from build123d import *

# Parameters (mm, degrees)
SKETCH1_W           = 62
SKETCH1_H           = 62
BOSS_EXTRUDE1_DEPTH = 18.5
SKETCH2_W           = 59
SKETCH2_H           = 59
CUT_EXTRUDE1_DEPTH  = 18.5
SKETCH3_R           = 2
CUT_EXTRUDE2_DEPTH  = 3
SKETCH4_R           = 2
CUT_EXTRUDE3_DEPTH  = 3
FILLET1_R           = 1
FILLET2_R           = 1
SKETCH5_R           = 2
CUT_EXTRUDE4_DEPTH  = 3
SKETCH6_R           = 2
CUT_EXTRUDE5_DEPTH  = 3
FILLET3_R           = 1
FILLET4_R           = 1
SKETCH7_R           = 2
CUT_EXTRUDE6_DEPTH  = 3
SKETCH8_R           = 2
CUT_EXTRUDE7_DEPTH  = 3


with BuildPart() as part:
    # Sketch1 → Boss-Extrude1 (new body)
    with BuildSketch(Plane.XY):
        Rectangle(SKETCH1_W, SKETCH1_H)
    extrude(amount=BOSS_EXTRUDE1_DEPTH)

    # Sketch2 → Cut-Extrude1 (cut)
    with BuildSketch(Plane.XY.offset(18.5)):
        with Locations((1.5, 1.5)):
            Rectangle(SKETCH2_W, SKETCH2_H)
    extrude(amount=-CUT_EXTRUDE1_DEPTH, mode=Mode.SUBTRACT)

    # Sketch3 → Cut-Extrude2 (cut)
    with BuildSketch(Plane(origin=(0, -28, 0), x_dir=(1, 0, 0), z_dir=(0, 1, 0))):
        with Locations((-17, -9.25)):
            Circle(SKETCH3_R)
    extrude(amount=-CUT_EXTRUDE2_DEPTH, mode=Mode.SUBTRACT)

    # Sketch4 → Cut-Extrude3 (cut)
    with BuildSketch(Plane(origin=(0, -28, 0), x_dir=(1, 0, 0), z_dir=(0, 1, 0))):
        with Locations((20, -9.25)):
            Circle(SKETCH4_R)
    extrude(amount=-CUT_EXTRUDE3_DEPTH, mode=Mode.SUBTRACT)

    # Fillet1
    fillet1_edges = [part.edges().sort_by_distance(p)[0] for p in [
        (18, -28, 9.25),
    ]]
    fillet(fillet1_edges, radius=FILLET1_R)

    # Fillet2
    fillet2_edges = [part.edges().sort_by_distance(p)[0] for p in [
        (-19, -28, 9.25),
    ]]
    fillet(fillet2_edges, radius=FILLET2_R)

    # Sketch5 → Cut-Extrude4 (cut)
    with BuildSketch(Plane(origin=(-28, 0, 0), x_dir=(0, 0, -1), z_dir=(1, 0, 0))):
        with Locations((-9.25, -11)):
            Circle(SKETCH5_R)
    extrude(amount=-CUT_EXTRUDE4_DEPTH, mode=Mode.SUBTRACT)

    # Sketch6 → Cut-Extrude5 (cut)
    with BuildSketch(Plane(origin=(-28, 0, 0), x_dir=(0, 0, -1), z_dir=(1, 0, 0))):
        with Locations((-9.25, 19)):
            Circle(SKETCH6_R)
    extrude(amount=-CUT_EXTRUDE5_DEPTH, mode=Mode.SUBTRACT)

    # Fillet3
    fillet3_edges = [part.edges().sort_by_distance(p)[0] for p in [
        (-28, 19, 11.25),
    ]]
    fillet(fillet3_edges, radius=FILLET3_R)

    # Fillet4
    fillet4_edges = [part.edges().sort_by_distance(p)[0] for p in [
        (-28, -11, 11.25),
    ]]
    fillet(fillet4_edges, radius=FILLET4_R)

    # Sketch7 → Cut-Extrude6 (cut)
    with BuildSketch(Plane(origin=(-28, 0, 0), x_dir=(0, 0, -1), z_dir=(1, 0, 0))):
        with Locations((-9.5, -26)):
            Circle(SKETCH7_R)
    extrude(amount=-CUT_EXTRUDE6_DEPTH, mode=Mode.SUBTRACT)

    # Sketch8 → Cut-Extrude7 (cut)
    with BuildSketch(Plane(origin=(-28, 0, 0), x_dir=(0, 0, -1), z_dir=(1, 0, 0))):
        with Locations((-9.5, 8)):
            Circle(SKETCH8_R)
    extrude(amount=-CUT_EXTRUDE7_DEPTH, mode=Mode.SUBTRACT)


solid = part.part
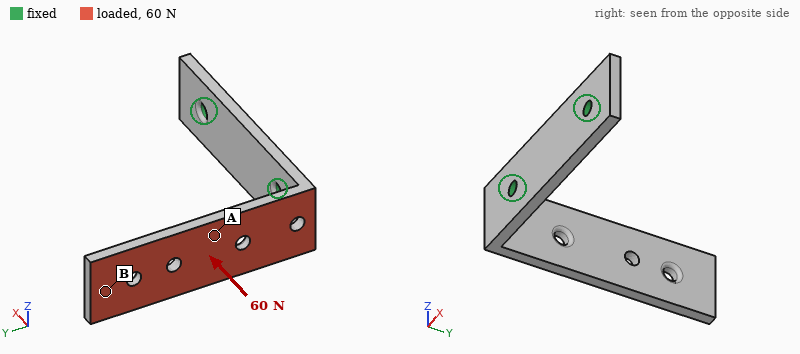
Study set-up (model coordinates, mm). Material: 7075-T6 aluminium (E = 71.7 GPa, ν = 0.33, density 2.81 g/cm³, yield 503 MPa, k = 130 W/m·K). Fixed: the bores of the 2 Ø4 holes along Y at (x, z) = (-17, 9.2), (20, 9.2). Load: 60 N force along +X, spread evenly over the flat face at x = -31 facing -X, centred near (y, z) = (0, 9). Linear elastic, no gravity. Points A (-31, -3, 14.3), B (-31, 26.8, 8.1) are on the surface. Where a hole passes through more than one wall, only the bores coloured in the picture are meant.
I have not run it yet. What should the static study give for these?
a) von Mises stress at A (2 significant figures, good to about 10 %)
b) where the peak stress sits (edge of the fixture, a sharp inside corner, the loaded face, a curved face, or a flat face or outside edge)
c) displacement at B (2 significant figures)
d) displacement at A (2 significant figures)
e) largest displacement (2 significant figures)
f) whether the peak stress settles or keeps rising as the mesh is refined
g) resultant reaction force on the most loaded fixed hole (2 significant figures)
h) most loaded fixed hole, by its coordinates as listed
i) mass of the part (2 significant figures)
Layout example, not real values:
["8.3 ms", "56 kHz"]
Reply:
["21 MPa", "edge of the fixture", "0.95 mm", "0.37 mm", "1.0 mm", "keeps rising", "42 N", "(20, 9.2)", "18 g"]
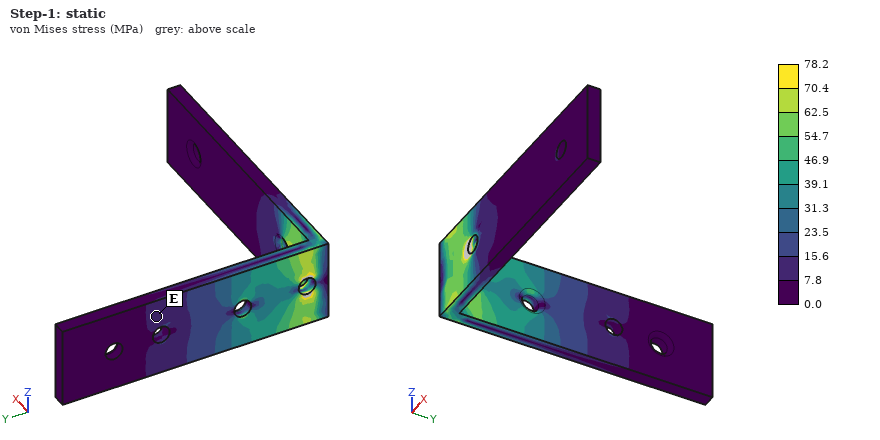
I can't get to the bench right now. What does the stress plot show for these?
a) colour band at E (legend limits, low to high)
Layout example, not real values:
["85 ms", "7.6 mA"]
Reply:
["7.8 to 15.6 MPa"]
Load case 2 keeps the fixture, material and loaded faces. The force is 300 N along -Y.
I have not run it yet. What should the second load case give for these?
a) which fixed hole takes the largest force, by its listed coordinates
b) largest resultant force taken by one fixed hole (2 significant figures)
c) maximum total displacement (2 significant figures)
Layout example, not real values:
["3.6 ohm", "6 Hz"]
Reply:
["(-17, 9.2)", "330 N", "0.83 mm"]
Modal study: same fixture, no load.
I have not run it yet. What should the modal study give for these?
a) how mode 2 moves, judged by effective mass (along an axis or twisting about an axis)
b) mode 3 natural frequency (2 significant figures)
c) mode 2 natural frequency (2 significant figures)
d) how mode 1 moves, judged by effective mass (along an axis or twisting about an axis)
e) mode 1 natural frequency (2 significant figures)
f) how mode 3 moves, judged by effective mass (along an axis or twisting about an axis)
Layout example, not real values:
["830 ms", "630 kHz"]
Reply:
["along Z", "3000 Hz", "900 Hz", "along X", "490 Hz", "along Y"]
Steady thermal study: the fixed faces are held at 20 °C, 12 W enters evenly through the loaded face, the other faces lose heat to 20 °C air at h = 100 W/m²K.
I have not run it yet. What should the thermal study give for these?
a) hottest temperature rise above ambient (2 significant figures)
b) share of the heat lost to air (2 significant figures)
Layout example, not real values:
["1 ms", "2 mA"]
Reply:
["39 K", "45 %"]
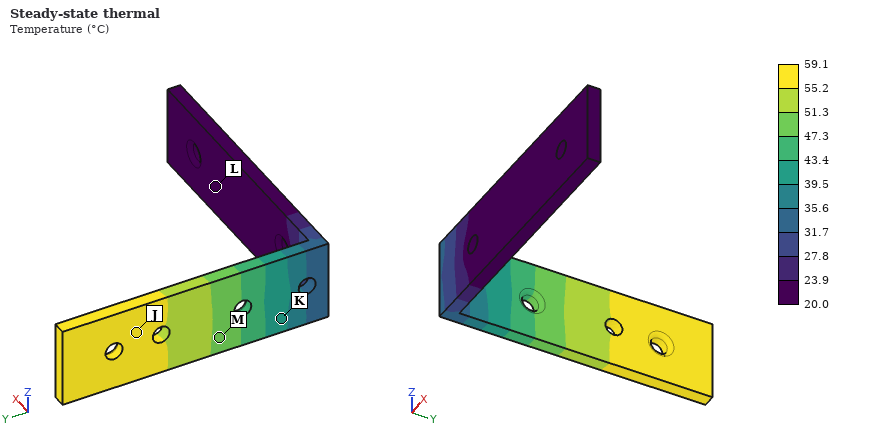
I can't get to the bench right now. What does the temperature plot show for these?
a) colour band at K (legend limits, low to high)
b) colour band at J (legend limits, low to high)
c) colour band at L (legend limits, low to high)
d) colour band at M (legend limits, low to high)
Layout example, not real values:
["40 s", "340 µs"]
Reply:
["39.5 to 43.4 °C", "55.2 to 59.1 °C", "20.0 to 23.9 °C", "47.3 to 51.3 °C"]
